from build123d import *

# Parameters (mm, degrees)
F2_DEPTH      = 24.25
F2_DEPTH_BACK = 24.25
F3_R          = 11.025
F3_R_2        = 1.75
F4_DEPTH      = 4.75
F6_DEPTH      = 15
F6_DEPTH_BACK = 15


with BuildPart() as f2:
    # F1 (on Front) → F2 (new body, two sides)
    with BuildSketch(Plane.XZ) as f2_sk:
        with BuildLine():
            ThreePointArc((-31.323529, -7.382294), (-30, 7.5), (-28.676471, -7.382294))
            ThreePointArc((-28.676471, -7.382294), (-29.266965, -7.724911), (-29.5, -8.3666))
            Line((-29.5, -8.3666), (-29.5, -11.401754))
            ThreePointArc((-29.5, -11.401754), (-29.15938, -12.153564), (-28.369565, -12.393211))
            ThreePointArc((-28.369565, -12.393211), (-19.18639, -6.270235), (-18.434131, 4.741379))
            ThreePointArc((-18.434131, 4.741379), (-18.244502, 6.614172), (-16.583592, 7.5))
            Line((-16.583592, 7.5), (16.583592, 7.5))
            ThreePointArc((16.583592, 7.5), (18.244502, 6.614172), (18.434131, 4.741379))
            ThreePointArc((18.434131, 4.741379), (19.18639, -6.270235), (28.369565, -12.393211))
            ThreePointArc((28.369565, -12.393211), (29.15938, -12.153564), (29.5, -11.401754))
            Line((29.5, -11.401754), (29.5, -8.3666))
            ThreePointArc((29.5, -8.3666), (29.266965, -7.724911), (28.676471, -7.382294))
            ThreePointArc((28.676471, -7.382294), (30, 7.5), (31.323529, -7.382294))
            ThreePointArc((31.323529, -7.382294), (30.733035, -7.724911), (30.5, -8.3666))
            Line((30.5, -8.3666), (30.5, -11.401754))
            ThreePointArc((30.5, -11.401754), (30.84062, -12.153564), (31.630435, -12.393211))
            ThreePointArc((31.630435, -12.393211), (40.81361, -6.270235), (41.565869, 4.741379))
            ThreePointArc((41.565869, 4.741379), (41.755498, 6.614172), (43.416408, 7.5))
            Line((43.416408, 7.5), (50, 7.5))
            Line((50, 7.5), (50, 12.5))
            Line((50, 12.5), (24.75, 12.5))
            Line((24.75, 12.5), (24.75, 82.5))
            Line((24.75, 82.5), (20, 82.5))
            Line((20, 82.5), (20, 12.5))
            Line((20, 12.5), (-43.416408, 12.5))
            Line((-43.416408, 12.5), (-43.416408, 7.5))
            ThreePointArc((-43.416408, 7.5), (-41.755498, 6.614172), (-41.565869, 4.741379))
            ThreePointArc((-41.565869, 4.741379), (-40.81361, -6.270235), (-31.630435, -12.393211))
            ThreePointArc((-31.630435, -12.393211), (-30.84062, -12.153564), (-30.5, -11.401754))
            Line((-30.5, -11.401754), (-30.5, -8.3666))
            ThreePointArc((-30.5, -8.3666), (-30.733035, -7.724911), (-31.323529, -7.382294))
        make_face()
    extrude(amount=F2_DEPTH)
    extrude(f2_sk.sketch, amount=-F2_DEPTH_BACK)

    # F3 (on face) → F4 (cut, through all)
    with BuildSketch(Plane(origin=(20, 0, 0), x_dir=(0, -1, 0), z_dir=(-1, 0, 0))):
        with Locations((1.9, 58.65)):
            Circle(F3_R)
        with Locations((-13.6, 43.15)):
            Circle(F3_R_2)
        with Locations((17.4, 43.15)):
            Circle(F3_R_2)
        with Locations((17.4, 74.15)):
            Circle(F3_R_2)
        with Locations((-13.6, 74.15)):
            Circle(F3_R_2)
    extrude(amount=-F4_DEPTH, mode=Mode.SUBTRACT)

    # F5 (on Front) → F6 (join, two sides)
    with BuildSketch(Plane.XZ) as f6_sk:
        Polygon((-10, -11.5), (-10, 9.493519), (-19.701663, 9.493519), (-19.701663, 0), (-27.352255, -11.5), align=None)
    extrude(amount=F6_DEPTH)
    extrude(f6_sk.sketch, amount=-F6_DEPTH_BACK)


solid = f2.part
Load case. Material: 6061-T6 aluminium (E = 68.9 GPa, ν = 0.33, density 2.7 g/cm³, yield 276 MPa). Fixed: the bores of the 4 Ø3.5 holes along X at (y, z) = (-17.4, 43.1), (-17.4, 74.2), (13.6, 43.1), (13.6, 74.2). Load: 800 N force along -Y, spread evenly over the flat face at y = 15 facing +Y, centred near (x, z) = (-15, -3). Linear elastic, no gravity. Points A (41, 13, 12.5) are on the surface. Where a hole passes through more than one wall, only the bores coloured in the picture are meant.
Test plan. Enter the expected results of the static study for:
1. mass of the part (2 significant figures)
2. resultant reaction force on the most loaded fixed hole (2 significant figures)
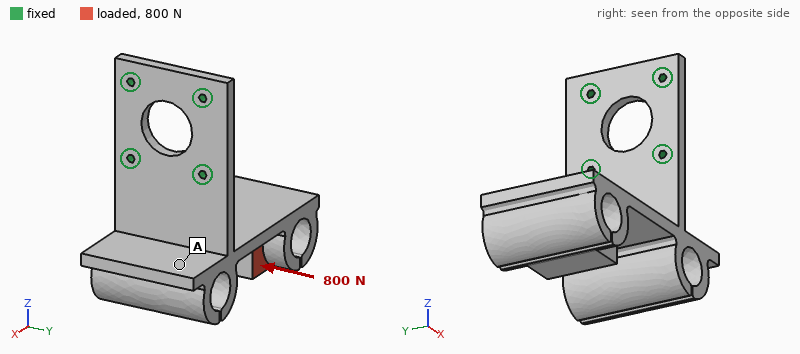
180 g
1.4 kN
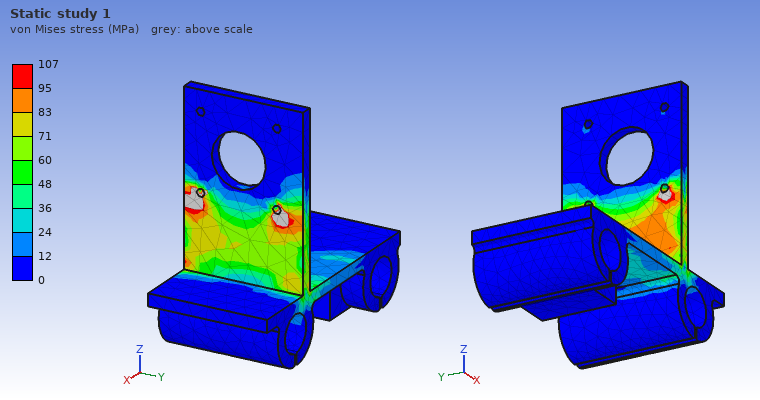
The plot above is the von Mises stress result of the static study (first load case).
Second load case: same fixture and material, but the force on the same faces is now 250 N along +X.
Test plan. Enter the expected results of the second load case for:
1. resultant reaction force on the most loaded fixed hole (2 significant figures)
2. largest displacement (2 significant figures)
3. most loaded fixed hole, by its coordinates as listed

300 N
0.76 mm
(13.6, 43.1)
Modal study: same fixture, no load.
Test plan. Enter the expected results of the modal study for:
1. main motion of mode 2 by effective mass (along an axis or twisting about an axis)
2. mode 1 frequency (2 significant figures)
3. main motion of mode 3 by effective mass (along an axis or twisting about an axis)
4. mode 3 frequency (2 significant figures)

along Y
270 Hz
along X
1000 Hz
